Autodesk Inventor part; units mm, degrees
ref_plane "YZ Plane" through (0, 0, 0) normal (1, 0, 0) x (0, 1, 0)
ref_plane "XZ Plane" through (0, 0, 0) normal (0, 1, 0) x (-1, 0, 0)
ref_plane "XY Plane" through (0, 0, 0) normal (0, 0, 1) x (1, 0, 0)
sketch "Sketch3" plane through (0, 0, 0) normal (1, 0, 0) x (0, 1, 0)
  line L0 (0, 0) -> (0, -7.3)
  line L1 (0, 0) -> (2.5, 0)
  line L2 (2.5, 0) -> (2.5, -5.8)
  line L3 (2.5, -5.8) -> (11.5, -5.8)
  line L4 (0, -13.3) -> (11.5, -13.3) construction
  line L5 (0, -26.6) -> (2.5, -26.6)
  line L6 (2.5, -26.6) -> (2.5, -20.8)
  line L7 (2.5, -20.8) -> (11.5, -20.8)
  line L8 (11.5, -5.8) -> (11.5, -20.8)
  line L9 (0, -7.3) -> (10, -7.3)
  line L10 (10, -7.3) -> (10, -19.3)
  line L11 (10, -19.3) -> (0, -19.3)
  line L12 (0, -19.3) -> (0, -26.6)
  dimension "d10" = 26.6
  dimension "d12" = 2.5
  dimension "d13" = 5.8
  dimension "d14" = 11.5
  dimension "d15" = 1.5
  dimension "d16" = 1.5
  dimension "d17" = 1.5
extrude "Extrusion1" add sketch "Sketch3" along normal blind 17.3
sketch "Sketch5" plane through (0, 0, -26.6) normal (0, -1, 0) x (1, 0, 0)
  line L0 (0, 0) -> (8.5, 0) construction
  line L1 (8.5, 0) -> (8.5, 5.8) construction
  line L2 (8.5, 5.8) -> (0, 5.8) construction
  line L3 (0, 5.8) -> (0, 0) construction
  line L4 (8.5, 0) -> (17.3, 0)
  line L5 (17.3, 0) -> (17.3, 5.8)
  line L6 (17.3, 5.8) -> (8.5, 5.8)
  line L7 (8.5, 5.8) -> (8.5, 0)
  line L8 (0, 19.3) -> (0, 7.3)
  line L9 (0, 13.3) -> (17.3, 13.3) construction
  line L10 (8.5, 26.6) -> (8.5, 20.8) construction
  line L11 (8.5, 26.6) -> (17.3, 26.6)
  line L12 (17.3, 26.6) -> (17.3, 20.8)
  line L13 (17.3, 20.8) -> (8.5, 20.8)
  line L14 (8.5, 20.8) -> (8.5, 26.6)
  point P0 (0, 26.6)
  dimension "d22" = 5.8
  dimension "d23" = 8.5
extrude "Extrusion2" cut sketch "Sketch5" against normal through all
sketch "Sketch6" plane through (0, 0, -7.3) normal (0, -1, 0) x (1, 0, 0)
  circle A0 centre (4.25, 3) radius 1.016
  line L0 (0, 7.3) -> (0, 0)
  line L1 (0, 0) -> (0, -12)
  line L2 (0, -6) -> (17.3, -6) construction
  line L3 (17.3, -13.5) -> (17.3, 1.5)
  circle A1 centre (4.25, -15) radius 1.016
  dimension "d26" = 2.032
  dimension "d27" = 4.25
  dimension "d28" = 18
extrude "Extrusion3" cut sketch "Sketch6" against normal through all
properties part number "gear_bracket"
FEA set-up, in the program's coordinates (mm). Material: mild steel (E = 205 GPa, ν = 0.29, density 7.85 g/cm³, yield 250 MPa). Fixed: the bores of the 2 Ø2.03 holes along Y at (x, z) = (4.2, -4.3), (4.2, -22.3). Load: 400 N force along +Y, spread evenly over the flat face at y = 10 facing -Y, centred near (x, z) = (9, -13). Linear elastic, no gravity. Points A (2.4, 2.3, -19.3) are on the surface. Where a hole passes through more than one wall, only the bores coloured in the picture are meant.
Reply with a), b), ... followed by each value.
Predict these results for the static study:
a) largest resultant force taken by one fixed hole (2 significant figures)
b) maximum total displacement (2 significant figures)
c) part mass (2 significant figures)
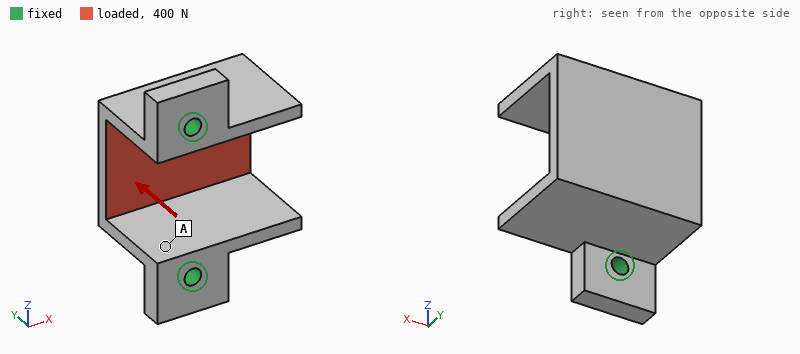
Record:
a) 210 N
b) 19 µm
c) 8.9 g
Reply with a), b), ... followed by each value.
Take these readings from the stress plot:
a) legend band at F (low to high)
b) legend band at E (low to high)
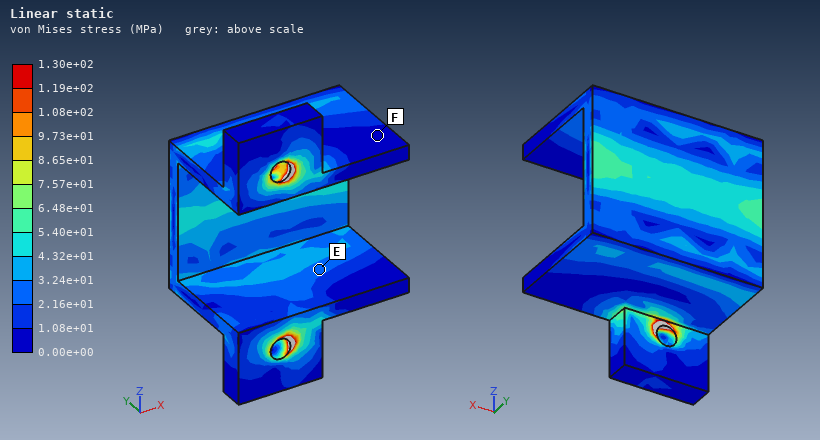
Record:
a) 0.00e+00 to 1.08e+01 MPa
b) 2.16e+01 to 3.24e+01 MPa
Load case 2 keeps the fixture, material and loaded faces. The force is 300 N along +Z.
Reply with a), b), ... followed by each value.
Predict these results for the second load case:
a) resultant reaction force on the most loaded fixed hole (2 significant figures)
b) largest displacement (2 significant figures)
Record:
a) 180 N
b) 24 µm
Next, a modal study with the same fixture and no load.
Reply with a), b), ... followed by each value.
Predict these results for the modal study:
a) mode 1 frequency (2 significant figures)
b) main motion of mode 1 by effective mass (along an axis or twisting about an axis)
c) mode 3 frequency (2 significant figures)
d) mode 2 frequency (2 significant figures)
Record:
a) 8700 Hz
b) along Z
c) 12 kHz
d) 9400 Hz
